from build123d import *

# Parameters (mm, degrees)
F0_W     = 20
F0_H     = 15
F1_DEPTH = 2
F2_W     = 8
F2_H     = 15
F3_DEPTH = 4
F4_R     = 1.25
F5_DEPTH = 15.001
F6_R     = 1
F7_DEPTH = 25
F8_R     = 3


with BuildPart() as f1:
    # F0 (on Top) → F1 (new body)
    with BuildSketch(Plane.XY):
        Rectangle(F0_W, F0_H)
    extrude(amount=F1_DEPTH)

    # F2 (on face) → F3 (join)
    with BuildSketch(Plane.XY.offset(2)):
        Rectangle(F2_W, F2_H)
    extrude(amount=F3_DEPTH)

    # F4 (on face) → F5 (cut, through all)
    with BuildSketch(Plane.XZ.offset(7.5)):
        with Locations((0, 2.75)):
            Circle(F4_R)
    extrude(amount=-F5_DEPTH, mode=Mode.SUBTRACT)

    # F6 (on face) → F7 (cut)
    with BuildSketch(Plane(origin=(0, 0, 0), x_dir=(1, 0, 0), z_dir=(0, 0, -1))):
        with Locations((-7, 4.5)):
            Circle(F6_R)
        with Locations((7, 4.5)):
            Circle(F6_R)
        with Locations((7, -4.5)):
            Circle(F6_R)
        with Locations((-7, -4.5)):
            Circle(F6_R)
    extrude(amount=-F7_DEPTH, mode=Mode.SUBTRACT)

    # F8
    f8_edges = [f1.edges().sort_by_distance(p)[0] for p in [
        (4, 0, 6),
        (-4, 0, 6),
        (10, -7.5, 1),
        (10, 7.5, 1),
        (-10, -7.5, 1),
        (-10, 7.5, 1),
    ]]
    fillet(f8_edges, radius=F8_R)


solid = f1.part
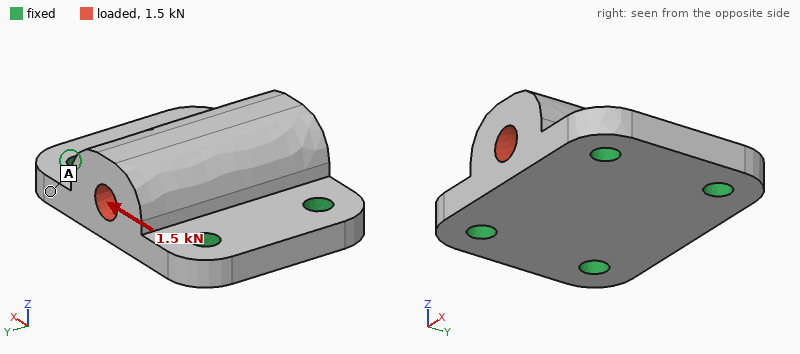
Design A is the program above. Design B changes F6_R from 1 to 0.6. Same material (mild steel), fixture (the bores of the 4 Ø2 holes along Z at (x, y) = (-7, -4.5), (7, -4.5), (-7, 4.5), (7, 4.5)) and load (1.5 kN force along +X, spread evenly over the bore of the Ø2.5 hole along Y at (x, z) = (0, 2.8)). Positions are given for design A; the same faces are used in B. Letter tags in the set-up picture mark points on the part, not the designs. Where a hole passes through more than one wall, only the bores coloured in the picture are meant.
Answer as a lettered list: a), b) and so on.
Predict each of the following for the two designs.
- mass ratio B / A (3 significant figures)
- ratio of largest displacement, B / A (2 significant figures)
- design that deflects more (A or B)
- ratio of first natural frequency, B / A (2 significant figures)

a) 1.02
b) 1.2
c) B
d) 0.86
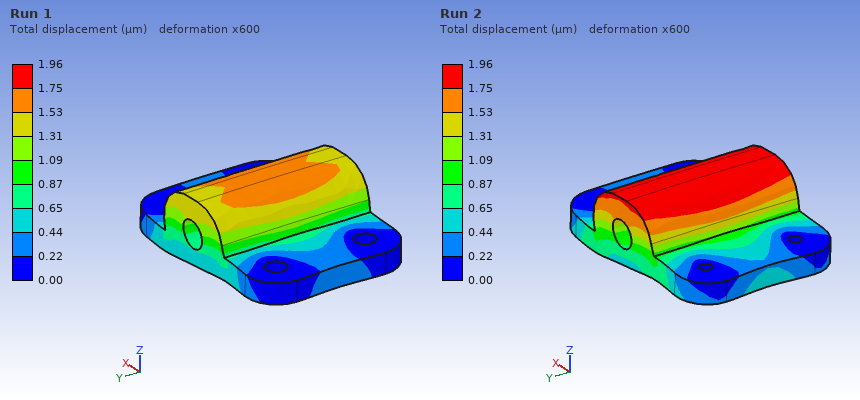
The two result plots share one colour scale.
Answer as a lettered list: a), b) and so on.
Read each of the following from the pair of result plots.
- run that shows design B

a) Run 2
